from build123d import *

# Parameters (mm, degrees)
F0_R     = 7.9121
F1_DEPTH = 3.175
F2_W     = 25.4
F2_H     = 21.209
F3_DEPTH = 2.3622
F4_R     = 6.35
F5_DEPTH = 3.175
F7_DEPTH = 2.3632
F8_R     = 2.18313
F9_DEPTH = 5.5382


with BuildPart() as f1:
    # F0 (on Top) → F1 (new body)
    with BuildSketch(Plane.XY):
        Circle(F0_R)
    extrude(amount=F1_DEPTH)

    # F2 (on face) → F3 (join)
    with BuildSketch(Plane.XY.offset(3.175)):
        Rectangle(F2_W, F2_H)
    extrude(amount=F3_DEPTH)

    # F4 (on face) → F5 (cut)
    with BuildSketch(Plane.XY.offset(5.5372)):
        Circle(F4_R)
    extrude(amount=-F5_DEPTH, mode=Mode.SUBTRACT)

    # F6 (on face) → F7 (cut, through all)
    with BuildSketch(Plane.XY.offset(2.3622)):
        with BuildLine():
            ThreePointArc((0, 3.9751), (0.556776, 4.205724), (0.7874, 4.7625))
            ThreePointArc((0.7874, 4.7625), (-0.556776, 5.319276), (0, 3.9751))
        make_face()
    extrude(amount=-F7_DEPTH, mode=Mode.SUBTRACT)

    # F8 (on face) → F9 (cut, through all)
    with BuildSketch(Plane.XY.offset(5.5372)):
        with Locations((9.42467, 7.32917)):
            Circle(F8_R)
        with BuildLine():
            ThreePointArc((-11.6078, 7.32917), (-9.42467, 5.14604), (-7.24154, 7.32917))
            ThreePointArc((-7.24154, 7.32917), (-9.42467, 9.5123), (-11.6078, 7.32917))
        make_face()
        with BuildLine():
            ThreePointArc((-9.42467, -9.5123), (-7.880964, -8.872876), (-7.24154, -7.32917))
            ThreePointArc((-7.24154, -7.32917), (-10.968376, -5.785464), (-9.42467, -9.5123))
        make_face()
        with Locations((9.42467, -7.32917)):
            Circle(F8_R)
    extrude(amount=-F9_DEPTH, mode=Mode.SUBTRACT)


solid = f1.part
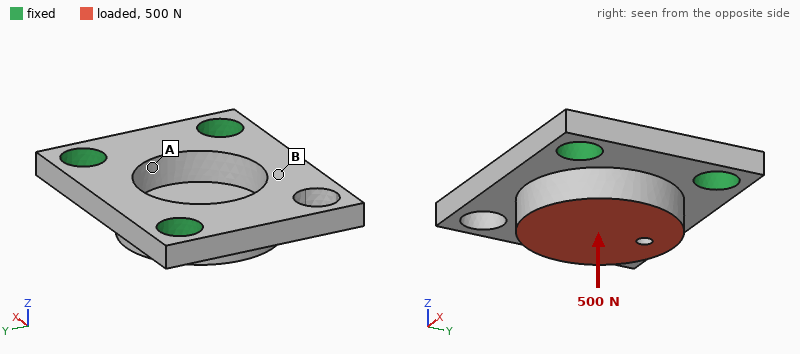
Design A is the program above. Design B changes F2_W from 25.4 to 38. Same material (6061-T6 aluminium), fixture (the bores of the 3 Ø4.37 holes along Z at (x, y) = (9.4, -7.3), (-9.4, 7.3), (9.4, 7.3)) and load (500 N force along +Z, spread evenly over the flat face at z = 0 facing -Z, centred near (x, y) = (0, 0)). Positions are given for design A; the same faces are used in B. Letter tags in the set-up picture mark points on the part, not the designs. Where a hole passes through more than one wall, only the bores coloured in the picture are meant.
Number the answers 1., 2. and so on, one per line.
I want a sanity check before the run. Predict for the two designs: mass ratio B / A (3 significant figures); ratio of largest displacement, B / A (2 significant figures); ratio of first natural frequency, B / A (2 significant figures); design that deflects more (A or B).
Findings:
1. 1.47
2. 0.84
3. 0.61
4. A
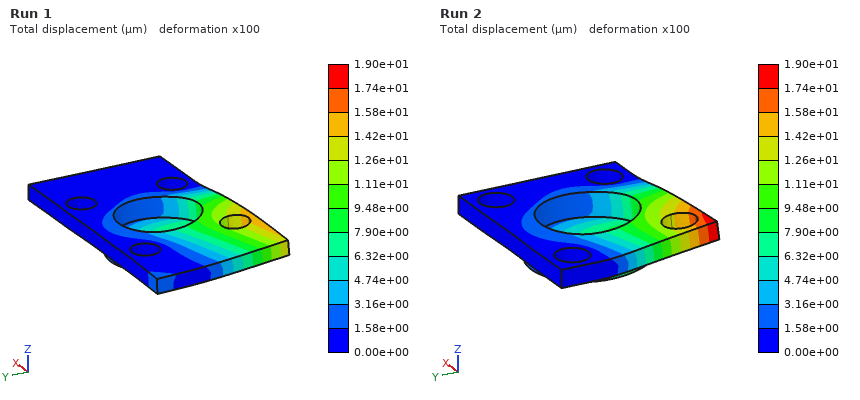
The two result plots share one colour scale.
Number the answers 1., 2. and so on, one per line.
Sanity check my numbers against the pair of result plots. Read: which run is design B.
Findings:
1. Run 1
